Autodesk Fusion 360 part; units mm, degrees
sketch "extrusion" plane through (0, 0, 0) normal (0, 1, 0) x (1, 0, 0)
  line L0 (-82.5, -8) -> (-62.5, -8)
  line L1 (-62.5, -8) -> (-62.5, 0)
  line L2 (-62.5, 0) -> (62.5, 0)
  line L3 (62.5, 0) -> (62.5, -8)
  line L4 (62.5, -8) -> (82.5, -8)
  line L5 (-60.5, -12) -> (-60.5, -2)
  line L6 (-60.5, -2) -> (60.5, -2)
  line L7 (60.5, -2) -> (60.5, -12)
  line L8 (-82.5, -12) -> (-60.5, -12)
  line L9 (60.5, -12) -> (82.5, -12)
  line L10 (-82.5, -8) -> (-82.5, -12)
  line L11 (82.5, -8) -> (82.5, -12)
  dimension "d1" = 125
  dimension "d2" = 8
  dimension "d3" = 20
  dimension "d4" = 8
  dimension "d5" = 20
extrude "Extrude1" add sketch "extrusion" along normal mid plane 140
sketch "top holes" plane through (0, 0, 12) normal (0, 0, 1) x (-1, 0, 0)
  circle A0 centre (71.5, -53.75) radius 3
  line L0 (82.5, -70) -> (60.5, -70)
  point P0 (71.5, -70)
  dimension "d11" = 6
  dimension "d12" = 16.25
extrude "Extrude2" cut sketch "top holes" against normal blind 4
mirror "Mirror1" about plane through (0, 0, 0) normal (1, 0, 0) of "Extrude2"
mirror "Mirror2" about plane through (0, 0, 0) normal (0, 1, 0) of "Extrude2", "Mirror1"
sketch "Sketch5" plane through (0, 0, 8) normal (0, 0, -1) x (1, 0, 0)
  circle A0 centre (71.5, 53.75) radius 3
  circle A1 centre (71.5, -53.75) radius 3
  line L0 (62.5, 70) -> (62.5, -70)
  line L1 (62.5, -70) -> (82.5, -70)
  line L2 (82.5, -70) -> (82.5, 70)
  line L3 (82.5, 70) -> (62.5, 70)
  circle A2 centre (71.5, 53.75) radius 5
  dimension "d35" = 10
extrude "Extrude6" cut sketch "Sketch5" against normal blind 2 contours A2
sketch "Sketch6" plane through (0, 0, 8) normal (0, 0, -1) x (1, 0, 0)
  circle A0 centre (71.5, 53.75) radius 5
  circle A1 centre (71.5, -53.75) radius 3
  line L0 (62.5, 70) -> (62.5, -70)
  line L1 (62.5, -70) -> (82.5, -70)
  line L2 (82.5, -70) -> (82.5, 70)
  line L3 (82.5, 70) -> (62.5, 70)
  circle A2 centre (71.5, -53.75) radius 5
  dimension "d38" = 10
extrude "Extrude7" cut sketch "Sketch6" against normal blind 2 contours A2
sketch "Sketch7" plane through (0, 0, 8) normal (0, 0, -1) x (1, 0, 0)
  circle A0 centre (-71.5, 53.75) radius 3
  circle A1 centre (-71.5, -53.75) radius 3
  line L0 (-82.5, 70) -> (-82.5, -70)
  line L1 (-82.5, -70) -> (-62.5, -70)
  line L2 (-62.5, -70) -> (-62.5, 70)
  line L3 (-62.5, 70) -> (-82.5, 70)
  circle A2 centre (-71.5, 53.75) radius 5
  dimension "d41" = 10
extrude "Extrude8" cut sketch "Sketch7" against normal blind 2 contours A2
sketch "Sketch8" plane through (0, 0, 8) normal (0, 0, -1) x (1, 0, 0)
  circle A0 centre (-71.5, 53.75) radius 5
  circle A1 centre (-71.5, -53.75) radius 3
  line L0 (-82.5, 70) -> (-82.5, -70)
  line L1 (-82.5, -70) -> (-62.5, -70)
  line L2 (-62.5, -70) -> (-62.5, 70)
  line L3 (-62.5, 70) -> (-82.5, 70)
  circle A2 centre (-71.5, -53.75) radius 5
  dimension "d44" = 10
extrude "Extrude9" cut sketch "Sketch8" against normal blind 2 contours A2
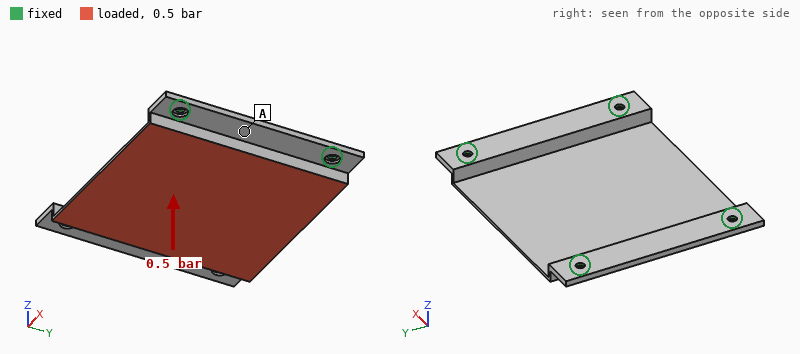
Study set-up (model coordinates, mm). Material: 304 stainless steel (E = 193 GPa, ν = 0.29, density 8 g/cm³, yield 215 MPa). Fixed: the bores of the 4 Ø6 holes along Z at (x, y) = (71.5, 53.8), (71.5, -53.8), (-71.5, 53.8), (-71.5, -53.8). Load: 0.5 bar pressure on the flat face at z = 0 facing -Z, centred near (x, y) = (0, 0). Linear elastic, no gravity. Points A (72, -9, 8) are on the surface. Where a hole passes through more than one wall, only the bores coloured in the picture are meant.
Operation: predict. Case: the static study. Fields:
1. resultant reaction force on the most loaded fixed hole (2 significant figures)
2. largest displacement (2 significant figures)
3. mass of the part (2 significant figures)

700 N
0.26 mm
500 g
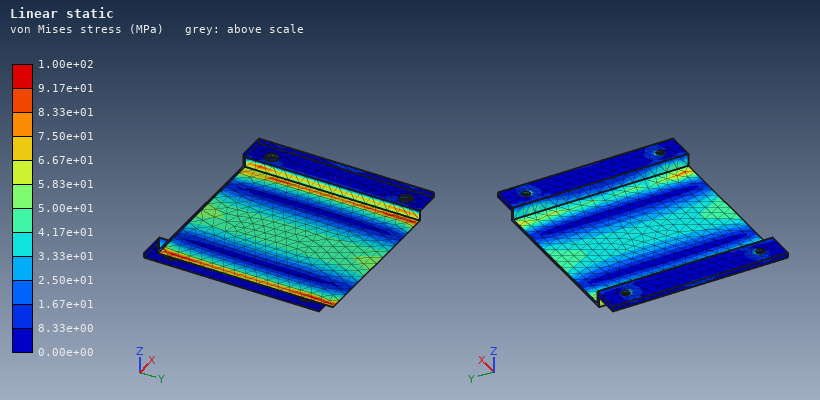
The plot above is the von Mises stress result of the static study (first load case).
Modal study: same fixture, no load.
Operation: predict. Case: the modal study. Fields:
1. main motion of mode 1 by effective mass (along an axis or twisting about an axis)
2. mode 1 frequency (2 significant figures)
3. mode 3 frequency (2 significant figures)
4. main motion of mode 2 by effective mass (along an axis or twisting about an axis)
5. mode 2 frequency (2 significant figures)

along Z
650 Hz
1100 Hz
twisting about X
770 Hz
